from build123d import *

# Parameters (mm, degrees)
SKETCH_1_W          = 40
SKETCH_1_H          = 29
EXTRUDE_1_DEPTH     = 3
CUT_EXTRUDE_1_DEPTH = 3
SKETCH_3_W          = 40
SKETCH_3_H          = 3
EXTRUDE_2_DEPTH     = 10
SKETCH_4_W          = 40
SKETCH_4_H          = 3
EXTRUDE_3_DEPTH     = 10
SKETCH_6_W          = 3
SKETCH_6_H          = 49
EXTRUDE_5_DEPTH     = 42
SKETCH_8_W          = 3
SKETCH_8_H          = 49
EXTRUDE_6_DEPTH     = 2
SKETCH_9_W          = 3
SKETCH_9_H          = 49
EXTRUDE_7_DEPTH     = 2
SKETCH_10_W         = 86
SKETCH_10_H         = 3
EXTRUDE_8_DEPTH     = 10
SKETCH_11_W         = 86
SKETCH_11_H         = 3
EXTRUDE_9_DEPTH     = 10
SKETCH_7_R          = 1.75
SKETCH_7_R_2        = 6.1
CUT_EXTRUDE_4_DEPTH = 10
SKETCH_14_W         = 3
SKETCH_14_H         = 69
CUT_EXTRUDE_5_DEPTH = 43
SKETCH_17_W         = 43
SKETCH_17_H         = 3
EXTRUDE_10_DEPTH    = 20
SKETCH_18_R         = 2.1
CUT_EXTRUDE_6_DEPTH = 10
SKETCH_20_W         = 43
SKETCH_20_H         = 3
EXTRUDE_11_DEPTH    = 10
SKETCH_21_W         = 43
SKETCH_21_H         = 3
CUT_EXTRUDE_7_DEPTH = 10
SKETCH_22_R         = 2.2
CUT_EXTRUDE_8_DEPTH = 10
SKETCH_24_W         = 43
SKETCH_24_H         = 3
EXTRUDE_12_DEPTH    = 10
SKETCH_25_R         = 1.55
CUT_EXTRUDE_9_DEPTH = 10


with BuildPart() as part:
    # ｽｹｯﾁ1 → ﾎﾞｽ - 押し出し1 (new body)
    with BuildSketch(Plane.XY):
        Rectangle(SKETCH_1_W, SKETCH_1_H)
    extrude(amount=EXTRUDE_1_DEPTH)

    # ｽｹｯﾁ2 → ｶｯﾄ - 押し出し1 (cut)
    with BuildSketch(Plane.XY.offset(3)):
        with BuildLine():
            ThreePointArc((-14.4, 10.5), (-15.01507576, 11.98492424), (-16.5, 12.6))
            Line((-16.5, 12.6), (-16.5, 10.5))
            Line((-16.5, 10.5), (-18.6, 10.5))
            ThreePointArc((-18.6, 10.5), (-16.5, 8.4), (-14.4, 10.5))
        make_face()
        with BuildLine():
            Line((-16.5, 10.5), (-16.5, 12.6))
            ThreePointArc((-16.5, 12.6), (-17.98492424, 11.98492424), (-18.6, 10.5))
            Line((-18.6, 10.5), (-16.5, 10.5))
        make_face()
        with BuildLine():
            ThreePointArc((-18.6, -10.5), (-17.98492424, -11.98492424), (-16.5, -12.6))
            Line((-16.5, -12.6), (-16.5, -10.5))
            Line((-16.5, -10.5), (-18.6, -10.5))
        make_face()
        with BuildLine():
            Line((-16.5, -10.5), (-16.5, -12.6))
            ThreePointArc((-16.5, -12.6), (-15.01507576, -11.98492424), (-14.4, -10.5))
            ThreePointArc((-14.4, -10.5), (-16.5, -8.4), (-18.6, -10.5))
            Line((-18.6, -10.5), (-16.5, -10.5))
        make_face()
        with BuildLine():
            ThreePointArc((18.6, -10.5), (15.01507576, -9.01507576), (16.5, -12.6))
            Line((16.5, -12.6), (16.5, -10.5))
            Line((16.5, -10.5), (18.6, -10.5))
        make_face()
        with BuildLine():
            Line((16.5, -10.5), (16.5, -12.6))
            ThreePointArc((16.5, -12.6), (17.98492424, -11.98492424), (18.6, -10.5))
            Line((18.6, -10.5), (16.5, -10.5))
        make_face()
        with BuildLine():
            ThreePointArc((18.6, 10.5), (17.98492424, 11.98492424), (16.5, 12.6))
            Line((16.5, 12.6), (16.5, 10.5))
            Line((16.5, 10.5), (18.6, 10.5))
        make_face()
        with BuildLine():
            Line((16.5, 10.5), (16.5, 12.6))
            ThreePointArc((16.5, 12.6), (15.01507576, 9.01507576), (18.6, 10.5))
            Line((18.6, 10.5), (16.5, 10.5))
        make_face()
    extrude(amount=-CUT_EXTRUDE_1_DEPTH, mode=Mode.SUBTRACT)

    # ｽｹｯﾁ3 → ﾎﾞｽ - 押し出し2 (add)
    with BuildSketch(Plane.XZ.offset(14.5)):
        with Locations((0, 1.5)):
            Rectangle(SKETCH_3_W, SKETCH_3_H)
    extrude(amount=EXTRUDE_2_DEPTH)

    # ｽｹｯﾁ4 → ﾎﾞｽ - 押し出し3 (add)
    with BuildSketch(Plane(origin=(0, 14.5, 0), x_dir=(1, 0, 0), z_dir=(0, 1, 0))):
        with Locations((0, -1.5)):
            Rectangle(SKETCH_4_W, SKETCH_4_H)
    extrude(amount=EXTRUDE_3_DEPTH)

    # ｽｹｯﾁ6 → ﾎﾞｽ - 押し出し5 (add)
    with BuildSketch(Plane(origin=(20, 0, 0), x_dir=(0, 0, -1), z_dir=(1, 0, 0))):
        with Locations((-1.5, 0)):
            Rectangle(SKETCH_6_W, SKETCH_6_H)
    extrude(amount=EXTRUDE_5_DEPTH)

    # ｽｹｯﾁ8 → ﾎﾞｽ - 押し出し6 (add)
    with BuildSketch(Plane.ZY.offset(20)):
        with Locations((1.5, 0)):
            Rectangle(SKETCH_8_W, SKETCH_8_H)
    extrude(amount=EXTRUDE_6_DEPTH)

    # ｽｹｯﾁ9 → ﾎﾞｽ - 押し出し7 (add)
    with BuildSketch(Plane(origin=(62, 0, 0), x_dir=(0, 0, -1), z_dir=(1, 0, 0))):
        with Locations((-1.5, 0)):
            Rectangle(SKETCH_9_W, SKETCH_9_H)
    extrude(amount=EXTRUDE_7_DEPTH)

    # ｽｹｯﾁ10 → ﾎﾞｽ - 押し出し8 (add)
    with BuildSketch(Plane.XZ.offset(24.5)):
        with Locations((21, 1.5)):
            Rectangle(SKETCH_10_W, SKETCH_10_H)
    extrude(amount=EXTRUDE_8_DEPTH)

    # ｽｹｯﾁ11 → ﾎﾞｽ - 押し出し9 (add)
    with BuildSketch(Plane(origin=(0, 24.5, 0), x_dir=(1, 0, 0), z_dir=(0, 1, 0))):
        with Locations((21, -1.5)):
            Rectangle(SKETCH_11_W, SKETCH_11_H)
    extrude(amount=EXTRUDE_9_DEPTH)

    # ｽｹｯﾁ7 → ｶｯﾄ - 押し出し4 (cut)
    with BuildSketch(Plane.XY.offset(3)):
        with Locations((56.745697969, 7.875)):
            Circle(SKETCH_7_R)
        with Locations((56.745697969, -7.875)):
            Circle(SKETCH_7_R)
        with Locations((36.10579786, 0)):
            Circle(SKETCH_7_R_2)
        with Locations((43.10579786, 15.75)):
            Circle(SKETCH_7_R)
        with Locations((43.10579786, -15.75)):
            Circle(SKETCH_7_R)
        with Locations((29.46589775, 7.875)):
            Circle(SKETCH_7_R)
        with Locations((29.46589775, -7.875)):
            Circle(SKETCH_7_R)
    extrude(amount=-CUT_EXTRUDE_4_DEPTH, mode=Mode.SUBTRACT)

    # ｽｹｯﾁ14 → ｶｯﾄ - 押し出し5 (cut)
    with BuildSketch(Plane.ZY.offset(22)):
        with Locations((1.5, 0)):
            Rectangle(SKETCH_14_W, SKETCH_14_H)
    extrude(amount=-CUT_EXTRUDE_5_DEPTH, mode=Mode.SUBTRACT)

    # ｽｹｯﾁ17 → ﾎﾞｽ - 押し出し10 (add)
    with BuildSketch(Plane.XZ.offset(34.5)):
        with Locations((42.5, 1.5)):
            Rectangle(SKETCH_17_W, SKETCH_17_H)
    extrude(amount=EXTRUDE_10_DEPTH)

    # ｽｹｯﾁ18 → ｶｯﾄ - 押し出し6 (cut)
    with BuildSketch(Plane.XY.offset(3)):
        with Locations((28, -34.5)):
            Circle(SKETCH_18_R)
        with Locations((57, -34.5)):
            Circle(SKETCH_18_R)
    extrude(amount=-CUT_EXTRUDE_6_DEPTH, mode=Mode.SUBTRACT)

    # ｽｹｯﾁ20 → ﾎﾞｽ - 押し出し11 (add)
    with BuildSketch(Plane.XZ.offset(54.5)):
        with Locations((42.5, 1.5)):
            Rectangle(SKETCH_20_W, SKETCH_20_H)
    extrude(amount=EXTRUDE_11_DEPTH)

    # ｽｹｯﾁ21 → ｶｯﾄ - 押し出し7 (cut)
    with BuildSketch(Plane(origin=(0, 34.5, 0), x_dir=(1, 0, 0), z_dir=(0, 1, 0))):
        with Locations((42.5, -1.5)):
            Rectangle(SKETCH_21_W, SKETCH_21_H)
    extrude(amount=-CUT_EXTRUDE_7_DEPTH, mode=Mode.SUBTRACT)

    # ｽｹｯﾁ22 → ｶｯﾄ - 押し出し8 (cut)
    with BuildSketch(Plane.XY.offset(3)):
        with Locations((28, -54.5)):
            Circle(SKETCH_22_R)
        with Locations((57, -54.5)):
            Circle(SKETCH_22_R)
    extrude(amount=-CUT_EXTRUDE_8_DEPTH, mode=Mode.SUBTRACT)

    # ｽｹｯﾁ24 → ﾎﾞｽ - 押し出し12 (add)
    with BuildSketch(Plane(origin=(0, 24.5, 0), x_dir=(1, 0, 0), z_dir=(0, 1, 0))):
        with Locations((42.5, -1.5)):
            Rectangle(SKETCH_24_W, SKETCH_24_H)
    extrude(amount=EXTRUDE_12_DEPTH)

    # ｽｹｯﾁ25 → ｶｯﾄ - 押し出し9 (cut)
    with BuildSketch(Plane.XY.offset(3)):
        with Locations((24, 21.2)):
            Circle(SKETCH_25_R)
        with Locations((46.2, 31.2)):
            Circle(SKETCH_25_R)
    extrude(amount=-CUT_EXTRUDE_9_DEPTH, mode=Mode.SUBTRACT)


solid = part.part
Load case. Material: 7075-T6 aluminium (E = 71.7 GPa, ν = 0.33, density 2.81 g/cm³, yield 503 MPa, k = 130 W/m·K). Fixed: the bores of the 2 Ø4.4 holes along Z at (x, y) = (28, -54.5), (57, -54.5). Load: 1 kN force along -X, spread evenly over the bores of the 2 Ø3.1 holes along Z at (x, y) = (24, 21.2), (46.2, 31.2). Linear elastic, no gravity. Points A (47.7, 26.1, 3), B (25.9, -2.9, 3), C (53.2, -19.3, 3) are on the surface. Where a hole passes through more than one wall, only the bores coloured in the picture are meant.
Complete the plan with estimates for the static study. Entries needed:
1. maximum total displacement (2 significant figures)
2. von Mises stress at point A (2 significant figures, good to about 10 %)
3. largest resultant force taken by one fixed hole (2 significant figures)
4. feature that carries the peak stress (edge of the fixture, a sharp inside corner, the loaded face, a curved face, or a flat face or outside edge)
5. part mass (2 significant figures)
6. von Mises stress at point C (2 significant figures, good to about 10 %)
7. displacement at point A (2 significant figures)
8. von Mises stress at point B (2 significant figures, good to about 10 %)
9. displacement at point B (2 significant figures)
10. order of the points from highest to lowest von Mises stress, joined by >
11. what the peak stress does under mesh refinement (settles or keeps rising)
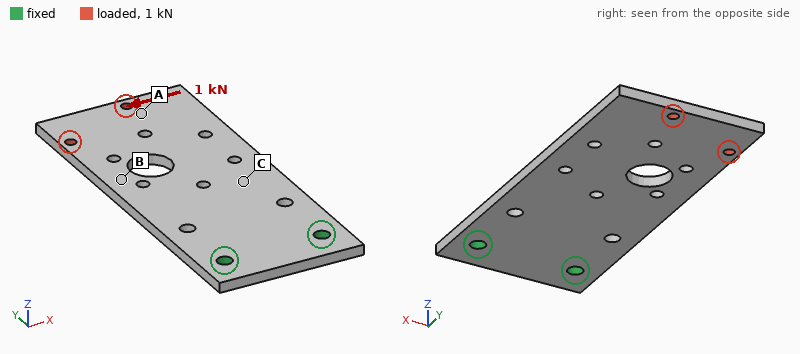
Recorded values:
0.21 mm
12 MPa
2.7 kN
edge of the fixture
34 g
26 MPa
0.18 mm
40 MPa
0.098 mm
B > C > A
keeps rising
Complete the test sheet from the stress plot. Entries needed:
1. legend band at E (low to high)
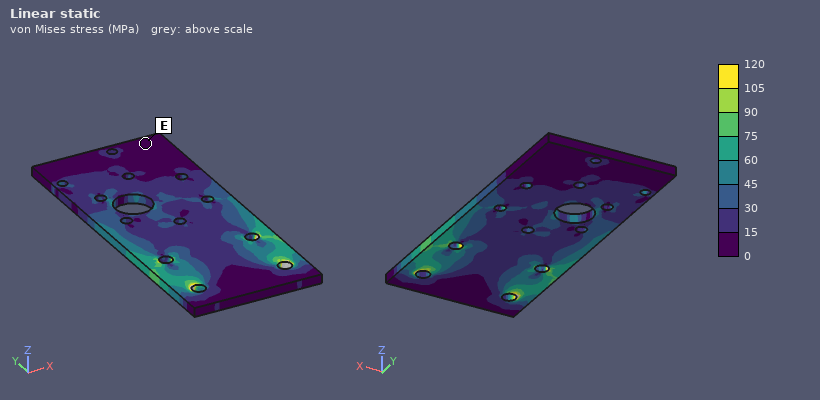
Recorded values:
0 to 15 MPa
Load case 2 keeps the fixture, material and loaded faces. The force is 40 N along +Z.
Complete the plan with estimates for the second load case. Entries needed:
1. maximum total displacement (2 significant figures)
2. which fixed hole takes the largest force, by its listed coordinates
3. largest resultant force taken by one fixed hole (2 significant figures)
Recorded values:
1.3 mm
(28, -54.5)
30 N
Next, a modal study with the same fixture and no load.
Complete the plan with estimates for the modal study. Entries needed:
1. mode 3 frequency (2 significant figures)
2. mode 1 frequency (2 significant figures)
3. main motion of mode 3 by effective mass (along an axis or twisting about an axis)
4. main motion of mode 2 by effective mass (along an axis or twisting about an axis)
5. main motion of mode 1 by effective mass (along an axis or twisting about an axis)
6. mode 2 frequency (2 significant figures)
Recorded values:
1900 Hz
310 Hz
along Z
twisting about Y
along Z
1300 Hz
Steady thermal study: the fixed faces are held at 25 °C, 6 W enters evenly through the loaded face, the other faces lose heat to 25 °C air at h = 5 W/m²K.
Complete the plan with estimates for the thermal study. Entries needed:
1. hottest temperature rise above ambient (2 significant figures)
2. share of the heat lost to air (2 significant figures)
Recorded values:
33 K
11 %
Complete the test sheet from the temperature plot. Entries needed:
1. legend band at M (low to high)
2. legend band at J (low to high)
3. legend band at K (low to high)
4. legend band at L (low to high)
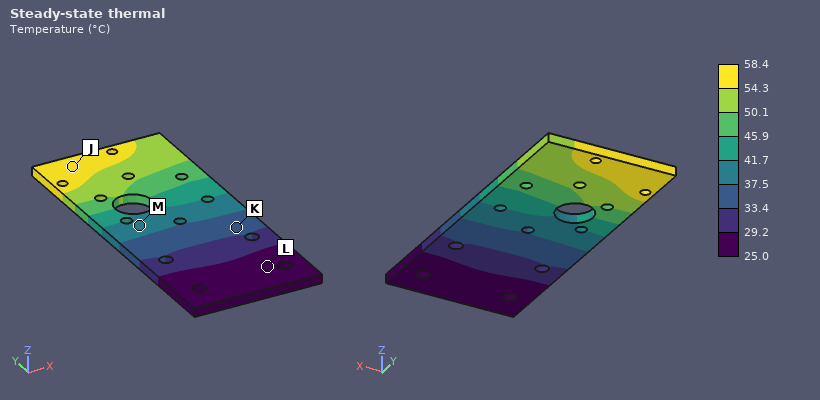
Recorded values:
37.5 to 41.7 °C
54.3 to 58.4 °C
33.4 to 37.5 °C
25.0 to 29.2 °C
